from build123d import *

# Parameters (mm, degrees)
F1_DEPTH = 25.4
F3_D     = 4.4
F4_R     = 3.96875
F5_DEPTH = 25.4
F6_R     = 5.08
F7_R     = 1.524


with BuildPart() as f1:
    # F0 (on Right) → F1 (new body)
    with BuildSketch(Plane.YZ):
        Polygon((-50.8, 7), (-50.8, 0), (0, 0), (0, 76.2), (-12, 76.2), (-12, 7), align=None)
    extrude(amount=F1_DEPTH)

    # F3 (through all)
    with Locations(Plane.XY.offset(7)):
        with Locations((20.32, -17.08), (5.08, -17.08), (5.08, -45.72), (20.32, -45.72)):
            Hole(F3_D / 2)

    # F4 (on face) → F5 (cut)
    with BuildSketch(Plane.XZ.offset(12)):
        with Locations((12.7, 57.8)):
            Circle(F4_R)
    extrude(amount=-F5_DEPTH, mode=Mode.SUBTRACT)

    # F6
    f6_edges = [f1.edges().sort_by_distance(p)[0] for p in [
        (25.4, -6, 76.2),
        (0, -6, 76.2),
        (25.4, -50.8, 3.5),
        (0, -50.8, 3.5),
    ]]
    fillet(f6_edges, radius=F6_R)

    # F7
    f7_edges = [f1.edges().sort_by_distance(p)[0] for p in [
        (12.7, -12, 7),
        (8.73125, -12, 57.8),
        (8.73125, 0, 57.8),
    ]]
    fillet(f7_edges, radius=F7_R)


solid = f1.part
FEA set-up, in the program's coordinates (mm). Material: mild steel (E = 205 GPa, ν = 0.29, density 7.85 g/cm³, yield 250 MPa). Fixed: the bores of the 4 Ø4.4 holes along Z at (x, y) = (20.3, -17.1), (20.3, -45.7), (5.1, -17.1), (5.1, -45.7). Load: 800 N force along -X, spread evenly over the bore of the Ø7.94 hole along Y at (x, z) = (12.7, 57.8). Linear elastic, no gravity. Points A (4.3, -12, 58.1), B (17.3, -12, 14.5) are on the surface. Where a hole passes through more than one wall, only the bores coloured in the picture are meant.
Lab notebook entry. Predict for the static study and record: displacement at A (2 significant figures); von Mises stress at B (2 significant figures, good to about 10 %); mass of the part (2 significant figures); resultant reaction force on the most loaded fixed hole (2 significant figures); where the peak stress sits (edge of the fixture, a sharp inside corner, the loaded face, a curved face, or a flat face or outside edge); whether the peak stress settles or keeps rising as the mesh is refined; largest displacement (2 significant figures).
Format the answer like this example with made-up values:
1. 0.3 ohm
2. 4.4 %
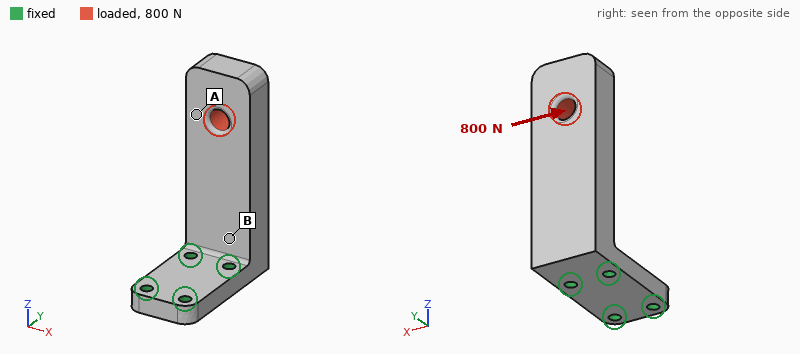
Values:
1. 43 µm
2. 25 MPa
3. 230 g
4. 2.3 kN
5. edge of the fixture
6. keeps rising
7. 59 µm
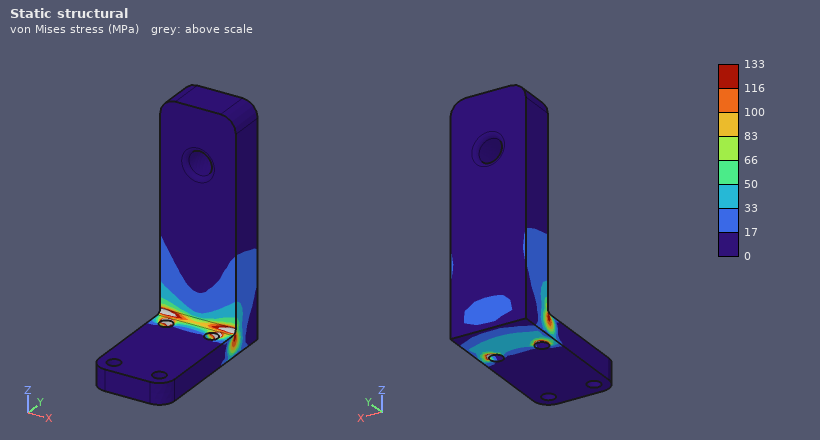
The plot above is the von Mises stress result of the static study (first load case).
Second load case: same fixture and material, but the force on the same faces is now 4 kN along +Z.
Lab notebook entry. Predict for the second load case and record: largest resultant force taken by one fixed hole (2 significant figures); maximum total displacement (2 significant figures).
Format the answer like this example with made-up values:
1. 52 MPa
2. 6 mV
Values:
1. 2.1 kN
2. 0.11 mm
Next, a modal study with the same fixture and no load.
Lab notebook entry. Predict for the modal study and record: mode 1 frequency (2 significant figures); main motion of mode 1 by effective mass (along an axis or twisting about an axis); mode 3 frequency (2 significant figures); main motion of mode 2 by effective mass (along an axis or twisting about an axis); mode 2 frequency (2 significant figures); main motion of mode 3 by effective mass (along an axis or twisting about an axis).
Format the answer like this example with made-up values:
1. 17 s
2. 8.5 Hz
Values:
1. 1100 Hz
2. along Y
3. 7300 Hz
4. along X
5. 2200 Hz
6. along Z
